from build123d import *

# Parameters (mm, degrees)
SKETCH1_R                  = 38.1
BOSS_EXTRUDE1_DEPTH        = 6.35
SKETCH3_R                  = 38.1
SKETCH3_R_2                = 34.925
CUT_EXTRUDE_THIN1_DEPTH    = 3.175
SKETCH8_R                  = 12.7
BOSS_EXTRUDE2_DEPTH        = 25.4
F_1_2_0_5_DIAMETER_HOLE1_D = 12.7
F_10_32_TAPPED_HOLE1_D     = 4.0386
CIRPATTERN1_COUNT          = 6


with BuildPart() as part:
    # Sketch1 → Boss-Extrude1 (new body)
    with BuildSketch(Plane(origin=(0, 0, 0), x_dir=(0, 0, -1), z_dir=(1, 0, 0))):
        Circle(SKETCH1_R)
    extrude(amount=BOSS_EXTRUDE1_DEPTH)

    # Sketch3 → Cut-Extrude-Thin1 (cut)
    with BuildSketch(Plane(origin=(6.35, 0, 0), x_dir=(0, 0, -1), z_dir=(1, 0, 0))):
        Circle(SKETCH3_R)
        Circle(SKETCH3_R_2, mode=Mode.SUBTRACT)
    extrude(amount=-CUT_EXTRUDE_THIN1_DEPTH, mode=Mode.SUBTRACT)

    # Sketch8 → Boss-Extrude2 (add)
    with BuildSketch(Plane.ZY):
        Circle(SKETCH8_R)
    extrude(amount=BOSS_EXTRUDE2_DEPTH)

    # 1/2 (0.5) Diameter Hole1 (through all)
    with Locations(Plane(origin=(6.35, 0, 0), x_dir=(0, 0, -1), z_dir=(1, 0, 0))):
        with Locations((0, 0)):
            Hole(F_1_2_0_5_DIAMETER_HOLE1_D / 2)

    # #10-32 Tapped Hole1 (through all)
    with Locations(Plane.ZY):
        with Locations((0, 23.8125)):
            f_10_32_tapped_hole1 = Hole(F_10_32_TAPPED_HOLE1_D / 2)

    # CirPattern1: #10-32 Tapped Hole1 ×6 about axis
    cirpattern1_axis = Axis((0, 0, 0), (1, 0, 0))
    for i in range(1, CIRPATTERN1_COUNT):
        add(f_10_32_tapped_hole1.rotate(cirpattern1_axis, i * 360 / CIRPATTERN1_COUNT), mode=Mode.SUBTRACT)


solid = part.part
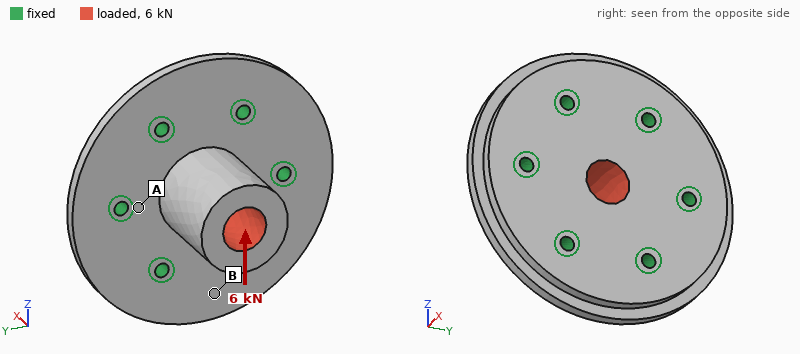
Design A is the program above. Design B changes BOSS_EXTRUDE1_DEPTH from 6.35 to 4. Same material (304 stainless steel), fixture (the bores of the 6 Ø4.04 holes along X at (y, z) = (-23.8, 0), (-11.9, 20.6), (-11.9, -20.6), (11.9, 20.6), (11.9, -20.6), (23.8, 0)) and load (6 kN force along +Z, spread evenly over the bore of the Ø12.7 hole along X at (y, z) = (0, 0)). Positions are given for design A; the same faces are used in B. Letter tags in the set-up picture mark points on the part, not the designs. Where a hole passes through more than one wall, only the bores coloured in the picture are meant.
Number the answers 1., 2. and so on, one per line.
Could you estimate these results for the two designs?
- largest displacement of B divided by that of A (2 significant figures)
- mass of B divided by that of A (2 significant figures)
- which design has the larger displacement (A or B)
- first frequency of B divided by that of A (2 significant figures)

1. 2.0
2. 0.76
3. B
4. 0.74
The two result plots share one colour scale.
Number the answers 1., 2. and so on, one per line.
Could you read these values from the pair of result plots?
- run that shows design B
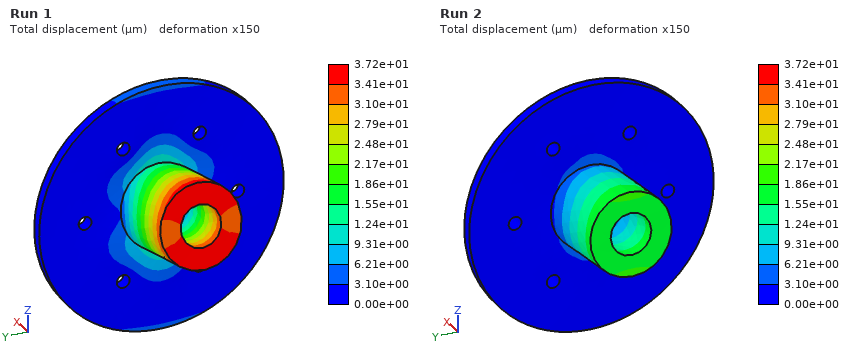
1. Run 1
